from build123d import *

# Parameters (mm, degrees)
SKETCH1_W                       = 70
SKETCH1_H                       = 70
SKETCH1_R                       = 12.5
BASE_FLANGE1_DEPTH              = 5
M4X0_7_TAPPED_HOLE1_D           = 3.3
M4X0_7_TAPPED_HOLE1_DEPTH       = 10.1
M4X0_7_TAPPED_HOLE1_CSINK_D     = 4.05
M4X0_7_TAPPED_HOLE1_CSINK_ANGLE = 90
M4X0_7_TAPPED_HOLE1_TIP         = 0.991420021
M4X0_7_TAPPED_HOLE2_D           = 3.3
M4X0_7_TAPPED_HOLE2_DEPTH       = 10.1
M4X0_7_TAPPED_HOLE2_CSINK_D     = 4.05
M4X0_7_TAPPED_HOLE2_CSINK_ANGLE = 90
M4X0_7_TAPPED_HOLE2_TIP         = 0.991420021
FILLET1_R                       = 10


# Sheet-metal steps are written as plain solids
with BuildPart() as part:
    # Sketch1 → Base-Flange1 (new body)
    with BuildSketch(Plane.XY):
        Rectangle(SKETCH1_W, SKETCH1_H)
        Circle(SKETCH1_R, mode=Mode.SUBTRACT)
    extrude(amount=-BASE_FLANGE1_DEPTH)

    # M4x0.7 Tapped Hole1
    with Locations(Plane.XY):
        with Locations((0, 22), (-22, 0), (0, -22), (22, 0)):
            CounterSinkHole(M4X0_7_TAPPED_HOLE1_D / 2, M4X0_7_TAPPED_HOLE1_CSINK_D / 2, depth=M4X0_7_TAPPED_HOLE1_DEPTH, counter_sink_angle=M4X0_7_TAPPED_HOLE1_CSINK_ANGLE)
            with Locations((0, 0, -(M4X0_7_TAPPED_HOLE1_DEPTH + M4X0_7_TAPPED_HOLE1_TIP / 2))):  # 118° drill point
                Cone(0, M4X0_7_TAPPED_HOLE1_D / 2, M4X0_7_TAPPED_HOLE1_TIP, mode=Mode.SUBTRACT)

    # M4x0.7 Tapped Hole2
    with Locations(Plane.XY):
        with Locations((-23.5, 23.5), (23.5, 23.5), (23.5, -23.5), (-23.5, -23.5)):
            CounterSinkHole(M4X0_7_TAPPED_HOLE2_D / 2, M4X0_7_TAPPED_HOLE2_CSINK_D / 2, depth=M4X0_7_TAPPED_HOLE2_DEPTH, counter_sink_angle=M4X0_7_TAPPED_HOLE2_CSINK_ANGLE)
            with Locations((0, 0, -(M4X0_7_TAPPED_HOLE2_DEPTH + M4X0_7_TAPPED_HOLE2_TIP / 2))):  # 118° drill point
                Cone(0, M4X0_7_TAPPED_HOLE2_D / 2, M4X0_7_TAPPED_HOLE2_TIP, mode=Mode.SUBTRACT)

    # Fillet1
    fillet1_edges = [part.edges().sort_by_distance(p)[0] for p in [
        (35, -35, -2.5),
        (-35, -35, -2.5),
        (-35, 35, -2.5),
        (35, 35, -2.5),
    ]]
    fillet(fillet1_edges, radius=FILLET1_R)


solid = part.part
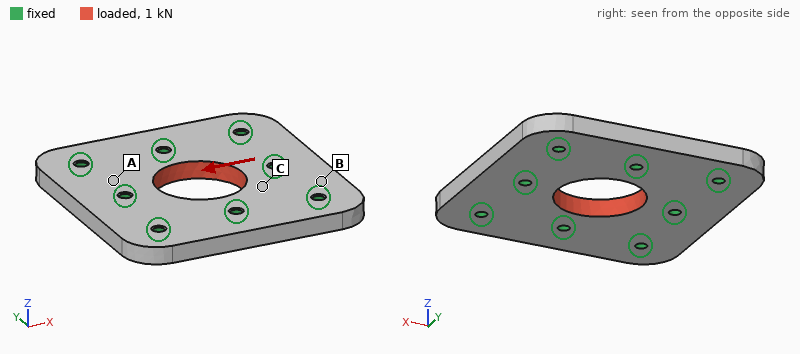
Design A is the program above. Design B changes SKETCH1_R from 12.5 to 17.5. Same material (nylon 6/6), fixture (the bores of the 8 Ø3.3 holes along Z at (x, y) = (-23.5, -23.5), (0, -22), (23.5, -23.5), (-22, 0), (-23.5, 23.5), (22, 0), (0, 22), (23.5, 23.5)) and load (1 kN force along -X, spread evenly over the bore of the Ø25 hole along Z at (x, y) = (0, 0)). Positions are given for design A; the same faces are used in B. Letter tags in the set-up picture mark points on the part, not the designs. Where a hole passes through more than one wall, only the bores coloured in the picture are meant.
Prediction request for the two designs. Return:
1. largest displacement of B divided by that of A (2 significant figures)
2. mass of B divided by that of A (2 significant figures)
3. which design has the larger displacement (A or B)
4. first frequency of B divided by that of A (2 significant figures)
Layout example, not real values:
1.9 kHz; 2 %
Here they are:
0.69; 0.89; A; 0.99
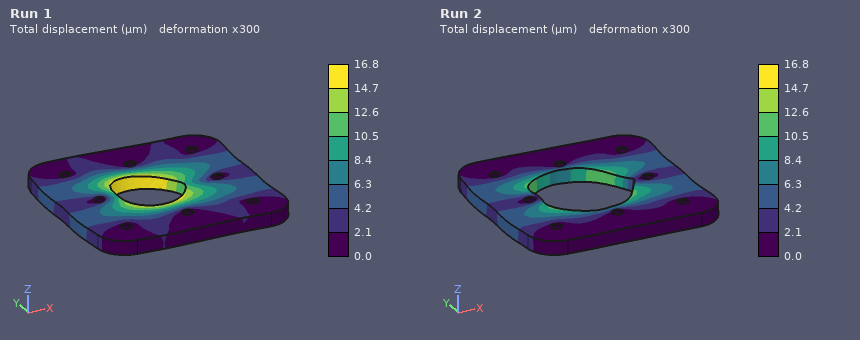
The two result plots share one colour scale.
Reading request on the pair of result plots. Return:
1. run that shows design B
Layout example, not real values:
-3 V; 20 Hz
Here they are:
Run 2
